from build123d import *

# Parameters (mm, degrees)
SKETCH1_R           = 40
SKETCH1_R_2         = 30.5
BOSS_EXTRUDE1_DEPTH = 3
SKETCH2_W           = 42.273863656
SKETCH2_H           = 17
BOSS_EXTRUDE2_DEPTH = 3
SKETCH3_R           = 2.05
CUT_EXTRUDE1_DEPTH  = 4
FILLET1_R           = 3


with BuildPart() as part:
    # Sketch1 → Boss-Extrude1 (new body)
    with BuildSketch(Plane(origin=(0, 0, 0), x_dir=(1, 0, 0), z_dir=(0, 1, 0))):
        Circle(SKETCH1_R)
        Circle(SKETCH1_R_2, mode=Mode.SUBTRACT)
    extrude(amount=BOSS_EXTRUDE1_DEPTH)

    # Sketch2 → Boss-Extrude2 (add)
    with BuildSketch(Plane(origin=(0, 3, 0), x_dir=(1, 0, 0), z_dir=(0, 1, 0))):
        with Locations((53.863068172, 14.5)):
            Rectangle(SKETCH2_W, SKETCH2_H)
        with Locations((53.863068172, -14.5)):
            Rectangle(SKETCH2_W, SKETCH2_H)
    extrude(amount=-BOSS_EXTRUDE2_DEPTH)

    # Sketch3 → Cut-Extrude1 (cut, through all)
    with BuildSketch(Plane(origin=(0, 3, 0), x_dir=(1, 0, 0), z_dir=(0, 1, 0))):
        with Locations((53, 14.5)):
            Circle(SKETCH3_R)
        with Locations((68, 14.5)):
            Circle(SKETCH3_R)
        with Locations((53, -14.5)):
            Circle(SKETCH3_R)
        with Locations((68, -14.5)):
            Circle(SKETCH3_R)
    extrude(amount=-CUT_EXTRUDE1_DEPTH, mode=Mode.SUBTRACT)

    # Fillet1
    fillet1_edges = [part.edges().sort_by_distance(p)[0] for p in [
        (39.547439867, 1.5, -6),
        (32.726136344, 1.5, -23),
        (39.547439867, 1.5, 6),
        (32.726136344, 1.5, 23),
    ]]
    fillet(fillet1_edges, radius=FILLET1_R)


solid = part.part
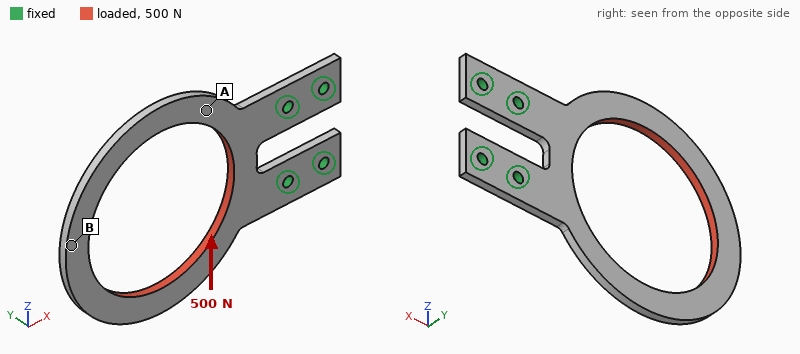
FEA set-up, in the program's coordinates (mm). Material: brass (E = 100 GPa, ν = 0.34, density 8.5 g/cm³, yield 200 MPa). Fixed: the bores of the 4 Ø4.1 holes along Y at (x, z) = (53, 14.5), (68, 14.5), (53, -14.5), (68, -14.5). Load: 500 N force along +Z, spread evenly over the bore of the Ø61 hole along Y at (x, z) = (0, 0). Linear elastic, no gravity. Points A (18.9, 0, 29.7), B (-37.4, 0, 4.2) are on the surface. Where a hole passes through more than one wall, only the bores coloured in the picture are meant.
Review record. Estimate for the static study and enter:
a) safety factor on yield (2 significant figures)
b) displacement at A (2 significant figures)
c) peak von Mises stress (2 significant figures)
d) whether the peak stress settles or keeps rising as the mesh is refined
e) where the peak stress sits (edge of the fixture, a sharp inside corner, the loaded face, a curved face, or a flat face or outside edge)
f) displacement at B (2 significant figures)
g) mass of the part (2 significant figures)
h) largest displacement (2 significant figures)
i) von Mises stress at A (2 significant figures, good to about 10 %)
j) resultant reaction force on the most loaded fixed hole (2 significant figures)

1.2
0.065 mm
170 MPa
settles
a curved face
0.27 mm
85 g
0.27 mm
19 MPa
670 N
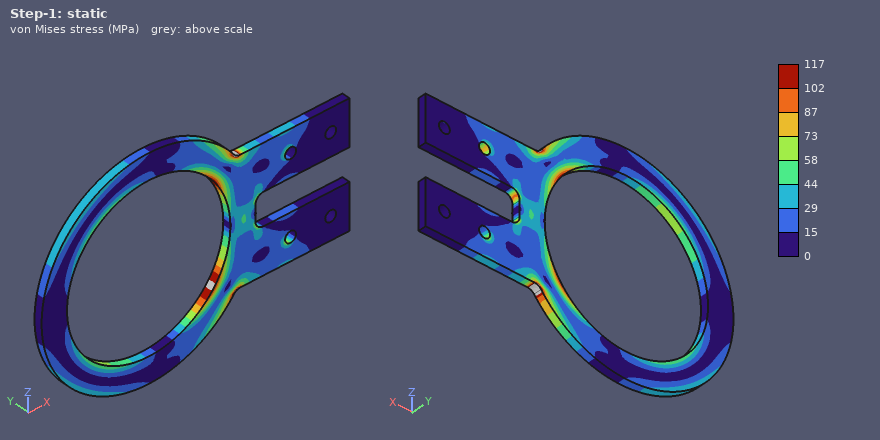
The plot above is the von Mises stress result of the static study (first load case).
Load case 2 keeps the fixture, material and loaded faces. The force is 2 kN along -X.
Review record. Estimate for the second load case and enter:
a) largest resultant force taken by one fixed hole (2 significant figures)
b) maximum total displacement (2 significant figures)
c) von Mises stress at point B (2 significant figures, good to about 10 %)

920 N
0.14 mm
40 MPa
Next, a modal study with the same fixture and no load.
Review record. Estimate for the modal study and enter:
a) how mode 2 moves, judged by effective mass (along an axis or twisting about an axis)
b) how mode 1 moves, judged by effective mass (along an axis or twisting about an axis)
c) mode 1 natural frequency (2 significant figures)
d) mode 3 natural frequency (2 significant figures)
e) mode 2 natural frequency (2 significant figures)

twisting about X
along Y
180 Hz
950 Hz
430 Hz
